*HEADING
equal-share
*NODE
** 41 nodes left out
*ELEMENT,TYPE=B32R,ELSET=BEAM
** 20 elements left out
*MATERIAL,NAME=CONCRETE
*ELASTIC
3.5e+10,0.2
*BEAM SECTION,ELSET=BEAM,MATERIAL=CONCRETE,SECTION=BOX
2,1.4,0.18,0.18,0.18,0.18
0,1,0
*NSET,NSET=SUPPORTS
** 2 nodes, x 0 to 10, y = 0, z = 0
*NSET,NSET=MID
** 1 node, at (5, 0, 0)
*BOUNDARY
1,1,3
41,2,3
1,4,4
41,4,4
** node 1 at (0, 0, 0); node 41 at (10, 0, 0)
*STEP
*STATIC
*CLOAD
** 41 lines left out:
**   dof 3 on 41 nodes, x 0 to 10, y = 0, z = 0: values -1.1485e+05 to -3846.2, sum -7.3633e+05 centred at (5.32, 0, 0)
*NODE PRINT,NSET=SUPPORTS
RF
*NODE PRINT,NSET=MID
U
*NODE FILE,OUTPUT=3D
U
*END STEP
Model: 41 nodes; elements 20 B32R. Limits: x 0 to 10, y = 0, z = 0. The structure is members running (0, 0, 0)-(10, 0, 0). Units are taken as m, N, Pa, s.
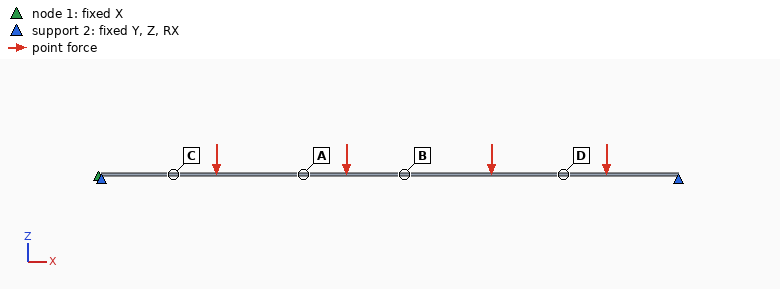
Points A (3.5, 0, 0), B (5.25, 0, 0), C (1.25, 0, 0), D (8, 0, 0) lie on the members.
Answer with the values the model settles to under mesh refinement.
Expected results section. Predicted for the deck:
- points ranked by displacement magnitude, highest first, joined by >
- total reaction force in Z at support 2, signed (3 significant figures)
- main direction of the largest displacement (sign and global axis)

B > A > D > C
7.36e+05 N
-Z
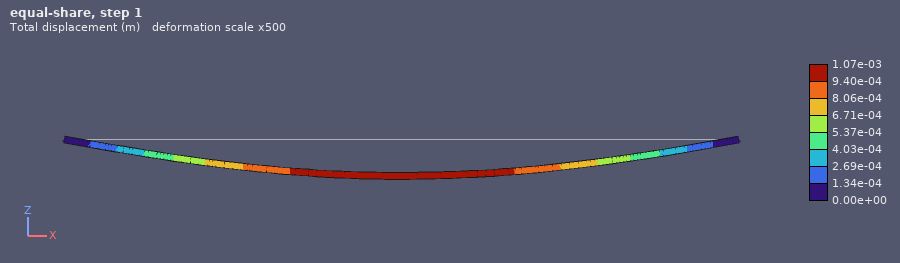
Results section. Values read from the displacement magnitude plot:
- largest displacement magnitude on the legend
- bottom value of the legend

1.07e-03 m
0.00e+00 m
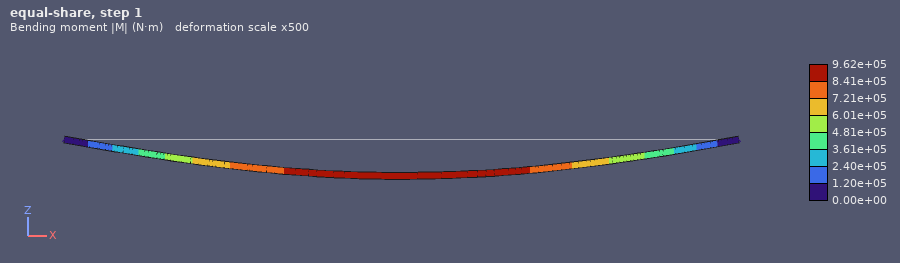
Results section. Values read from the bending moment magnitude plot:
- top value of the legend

9.62e+05 N·m
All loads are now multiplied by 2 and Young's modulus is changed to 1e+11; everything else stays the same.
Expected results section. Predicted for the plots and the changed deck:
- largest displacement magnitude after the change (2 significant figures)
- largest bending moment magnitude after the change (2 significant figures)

7.5e-04 m
1.9e+06 N·m
